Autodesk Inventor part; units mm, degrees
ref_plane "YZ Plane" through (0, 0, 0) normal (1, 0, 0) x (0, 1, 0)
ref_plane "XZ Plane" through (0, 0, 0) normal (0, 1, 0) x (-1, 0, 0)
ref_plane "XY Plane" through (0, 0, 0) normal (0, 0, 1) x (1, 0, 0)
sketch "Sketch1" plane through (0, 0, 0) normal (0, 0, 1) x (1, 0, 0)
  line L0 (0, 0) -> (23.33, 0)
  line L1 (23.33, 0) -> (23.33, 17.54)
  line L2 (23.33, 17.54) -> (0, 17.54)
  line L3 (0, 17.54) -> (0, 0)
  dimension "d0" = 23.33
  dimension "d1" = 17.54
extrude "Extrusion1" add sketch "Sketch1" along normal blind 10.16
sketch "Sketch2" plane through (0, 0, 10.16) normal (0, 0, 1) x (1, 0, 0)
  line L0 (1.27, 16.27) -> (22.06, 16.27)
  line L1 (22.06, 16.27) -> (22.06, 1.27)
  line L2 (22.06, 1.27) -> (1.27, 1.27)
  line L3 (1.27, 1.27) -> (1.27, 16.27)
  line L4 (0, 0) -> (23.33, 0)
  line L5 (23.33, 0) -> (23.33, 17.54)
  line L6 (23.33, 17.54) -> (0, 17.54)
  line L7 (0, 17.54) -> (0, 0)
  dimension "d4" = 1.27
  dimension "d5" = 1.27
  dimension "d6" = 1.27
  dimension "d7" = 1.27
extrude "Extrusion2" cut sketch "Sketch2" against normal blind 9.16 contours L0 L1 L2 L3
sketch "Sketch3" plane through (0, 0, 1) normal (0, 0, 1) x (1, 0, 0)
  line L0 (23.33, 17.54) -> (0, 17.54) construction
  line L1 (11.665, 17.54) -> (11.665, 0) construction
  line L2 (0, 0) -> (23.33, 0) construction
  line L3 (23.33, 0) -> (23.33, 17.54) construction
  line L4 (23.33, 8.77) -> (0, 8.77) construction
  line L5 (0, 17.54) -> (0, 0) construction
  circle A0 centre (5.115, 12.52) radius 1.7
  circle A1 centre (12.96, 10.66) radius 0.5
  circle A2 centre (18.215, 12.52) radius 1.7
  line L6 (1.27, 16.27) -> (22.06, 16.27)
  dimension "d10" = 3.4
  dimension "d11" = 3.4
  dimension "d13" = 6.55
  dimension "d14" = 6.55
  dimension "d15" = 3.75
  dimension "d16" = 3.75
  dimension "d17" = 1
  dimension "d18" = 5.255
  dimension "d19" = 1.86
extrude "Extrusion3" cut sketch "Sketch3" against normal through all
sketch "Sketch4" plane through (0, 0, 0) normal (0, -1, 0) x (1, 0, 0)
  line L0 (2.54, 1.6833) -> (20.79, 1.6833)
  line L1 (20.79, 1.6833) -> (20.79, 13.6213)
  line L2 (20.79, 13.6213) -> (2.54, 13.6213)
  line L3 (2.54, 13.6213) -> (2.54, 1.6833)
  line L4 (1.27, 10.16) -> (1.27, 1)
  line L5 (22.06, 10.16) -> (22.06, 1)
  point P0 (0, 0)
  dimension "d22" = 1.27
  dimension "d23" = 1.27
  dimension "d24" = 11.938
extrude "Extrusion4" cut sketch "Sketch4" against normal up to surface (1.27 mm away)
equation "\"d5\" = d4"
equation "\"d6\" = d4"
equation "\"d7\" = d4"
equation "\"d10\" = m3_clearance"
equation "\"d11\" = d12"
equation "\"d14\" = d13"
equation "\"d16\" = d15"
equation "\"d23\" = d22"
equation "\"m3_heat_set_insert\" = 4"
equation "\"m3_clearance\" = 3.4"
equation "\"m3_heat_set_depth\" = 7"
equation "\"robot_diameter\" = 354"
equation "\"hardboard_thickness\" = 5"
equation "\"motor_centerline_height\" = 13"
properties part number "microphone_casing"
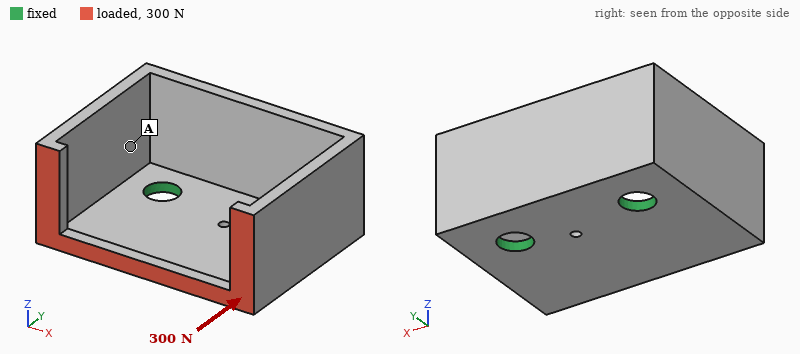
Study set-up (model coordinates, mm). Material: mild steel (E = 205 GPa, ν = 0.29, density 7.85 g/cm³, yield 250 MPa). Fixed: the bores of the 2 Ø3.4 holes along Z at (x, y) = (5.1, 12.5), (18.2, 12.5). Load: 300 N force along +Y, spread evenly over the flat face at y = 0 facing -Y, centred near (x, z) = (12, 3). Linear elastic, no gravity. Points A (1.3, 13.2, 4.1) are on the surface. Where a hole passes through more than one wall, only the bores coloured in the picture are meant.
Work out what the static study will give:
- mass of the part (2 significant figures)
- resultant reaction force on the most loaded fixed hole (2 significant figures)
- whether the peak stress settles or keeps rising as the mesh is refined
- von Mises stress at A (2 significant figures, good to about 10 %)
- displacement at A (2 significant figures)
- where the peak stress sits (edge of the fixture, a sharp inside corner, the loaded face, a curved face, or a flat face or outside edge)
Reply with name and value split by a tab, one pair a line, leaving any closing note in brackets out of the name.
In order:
mass of the part	8.5 g
resultant reaction force on the most loaded fixed hole	150 N
whether the peak stress settles or keeps rising as the mesh is refined	keeps rising
von Mises stress at A	22 MPa
displacement at A	6.2 µm
where the peak stress sits	edge of the fixture
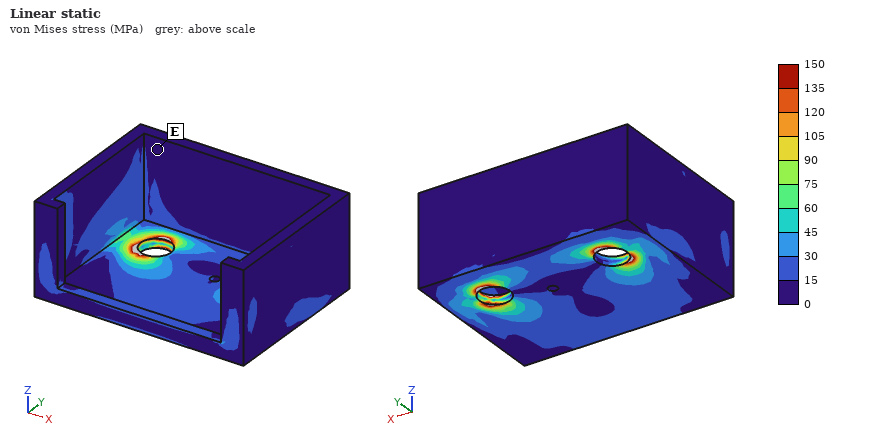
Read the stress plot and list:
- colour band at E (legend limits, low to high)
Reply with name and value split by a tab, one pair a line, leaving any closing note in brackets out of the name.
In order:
colour band at E	0 to 15 MPa
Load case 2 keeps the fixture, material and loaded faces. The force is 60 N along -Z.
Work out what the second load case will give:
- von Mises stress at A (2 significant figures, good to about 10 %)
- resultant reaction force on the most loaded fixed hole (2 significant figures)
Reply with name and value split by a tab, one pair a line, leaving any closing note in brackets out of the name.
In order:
von Mises stress at A	13 MPa
resultant reaction force on the most loaded fixed hole	30 N
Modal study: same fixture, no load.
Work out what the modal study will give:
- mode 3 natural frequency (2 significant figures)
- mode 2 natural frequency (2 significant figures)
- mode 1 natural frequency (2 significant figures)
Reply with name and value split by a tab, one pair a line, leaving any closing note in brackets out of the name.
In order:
mode 3 natural frequency	8700 Hz
mode 2 natural frequency	6700 Hz
mode 1 natural frequency	5400 Hz
